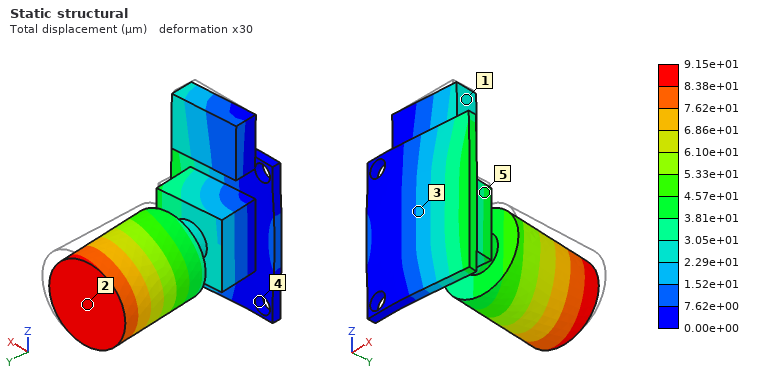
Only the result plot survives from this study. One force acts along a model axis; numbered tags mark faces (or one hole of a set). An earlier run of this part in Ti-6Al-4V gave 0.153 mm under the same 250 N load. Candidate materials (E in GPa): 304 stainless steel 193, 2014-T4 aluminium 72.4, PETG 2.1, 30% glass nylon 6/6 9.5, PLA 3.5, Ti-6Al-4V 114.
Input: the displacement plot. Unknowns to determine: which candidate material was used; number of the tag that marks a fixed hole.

304 stainless steel
4
